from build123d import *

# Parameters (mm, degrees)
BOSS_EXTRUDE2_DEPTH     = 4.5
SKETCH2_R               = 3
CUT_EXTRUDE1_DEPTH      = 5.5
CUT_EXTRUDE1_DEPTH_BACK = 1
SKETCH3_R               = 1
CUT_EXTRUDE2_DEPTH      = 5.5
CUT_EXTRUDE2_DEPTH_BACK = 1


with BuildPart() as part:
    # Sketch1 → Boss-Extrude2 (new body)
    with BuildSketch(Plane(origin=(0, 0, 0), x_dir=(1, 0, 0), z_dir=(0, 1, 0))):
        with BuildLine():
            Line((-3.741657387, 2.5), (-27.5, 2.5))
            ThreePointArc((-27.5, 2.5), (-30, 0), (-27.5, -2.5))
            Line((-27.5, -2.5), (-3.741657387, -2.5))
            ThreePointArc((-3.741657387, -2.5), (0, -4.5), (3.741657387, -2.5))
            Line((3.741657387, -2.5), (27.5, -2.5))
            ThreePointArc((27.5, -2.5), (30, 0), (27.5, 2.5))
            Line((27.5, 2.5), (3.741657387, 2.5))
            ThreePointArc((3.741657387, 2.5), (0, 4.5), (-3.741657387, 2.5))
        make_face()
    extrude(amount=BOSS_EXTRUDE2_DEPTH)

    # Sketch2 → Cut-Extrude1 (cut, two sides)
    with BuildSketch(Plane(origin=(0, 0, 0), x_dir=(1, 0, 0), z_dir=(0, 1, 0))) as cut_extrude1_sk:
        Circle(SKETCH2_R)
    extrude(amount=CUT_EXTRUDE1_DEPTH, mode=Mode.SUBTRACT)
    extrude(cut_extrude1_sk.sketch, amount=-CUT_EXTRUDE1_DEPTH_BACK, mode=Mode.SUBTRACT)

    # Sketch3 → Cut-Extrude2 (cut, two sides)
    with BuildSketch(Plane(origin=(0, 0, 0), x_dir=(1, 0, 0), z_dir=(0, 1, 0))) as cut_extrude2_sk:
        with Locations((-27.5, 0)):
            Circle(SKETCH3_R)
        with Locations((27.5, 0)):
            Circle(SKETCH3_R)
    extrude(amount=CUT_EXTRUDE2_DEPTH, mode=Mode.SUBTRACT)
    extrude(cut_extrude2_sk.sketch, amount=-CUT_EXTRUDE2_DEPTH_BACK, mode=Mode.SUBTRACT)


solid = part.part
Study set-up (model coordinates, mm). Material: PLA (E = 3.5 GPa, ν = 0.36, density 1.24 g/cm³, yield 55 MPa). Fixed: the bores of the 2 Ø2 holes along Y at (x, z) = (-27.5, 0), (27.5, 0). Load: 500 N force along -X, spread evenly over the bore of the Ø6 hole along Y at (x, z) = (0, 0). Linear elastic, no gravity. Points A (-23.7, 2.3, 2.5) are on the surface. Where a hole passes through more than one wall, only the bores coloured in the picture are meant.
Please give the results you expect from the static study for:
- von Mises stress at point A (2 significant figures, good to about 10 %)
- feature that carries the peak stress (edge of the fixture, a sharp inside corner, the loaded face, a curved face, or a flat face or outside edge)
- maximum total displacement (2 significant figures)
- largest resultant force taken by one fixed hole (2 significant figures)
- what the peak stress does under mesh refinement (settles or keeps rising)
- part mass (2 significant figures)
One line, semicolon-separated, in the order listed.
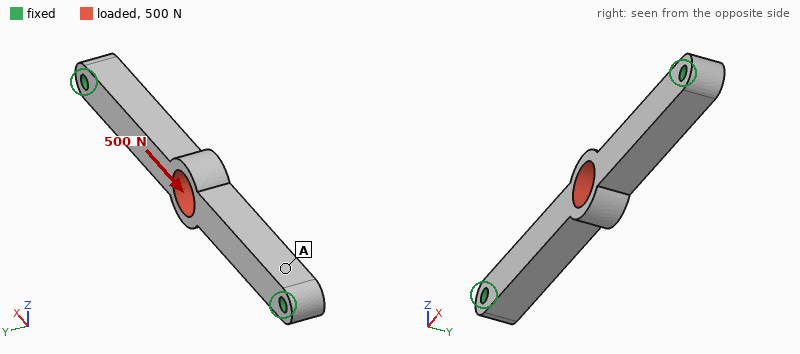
10 MPa; edge of the fixture; 96 µm; 250 N; keeps rising; 1.6 g
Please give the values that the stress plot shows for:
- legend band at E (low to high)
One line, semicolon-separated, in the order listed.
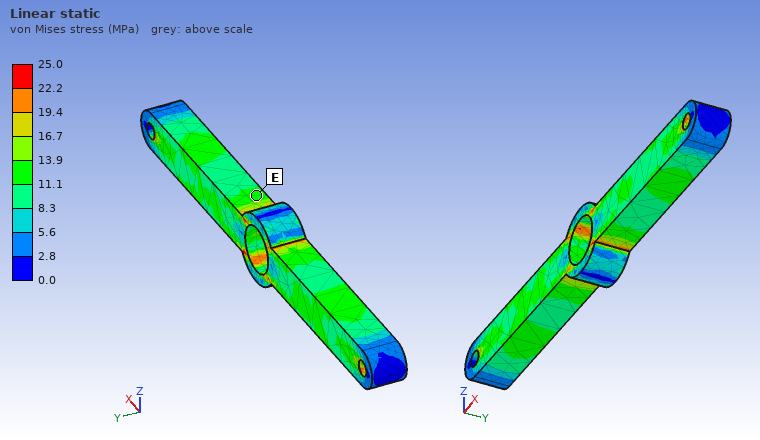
11.1 to 13.9 MPa
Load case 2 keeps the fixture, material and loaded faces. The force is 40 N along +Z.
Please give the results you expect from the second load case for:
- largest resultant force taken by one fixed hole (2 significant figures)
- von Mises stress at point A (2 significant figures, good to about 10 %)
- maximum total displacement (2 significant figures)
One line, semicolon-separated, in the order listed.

20 N; 10 MPa; 0.26 mm
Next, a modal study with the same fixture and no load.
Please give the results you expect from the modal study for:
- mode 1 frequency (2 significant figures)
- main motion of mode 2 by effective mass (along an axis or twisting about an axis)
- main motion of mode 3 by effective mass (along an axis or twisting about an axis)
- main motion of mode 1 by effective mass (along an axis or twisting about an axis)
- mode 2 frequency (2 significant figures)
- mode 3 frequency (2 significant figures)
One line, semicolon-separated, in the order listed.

2200 Hz; along Z; twisting about Y; along Y; 2500 Hz; 5600 Hz
